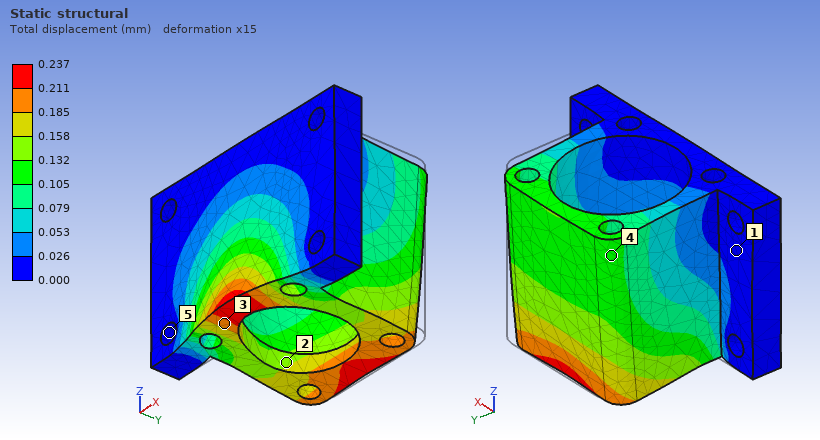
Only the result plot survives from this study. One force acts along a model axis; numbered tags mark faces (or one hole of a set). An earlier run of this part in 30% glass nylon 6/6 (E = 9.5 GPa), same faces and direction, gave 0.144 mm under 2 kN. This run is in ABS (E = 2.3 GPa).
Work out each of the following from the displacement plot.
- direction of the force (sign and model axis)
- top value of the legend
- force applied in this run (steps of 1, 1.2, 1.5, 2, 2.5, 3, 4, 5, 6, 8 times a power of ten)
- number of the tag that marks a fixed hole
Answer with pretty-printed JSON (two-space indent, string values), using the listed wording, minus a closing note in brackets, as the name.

{
  "direction of the force": "-Y",
  "top value of the legend": "0.237 mm",
  "force applied in this run": "800 N",
  "number of the tag that marks a fixed hole": "5"
}
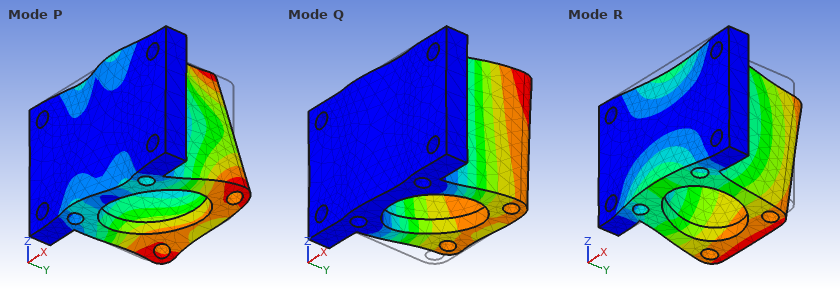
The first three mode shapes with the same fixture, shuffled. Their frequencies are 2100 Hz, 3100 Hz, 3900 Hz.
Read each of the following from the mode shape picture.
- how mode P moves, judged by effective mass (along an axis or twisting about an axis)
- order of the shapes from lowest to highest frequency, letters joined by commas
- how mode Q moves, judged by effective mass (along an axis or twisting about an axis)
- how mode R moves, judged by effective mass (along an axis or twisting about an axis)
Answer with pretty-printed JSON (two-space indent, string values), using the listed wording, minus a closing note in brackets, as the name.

{
  "how mode P moves, judged by effective mass": "twisting about Y",
  "order of the shapes from lowest to highest frequency, letters joined by commas": "Q, R, P",
  "how mode Q moves, judged by effective mass": "along X",
  "how mode R moves, judged by effective mass": "along Z"
}
